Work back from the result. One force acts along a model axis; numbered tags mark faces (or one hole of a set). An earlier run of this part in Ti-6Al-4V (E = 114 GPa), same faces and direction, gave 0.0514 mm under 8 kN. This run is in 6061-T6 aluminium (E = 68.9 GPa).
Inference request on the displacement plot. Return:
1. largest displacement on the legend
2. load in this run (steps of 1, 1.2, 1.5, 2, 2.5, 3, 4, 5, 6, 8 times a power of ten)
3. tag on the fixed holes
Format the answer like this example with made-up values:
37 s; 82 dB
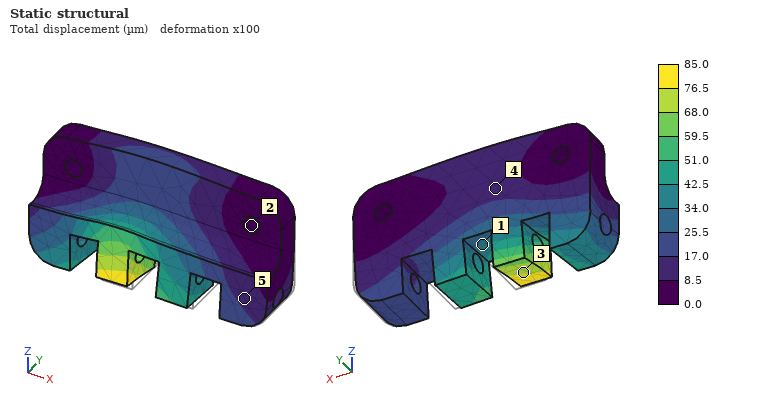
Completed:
85.0 µm; 8 kN; 2
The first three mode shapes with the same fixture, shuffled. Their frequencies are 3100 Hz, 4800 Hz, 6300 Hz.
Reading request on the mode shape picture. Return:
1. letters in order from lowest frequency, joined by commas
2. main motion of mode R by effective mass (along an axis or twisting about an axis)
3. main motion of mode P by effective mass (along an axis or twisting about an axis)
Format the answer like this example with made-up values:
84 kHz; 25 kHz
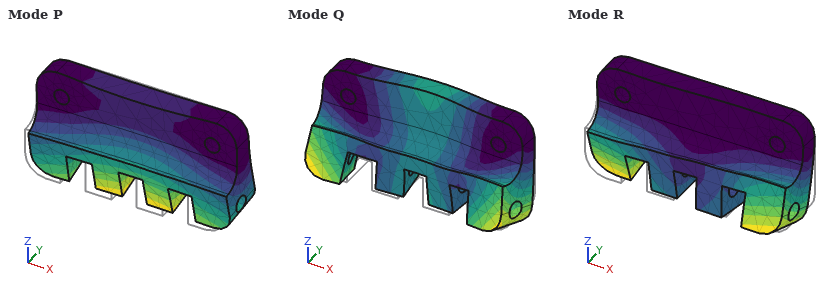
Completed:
P, R, Q; twisting about Z; along Y
